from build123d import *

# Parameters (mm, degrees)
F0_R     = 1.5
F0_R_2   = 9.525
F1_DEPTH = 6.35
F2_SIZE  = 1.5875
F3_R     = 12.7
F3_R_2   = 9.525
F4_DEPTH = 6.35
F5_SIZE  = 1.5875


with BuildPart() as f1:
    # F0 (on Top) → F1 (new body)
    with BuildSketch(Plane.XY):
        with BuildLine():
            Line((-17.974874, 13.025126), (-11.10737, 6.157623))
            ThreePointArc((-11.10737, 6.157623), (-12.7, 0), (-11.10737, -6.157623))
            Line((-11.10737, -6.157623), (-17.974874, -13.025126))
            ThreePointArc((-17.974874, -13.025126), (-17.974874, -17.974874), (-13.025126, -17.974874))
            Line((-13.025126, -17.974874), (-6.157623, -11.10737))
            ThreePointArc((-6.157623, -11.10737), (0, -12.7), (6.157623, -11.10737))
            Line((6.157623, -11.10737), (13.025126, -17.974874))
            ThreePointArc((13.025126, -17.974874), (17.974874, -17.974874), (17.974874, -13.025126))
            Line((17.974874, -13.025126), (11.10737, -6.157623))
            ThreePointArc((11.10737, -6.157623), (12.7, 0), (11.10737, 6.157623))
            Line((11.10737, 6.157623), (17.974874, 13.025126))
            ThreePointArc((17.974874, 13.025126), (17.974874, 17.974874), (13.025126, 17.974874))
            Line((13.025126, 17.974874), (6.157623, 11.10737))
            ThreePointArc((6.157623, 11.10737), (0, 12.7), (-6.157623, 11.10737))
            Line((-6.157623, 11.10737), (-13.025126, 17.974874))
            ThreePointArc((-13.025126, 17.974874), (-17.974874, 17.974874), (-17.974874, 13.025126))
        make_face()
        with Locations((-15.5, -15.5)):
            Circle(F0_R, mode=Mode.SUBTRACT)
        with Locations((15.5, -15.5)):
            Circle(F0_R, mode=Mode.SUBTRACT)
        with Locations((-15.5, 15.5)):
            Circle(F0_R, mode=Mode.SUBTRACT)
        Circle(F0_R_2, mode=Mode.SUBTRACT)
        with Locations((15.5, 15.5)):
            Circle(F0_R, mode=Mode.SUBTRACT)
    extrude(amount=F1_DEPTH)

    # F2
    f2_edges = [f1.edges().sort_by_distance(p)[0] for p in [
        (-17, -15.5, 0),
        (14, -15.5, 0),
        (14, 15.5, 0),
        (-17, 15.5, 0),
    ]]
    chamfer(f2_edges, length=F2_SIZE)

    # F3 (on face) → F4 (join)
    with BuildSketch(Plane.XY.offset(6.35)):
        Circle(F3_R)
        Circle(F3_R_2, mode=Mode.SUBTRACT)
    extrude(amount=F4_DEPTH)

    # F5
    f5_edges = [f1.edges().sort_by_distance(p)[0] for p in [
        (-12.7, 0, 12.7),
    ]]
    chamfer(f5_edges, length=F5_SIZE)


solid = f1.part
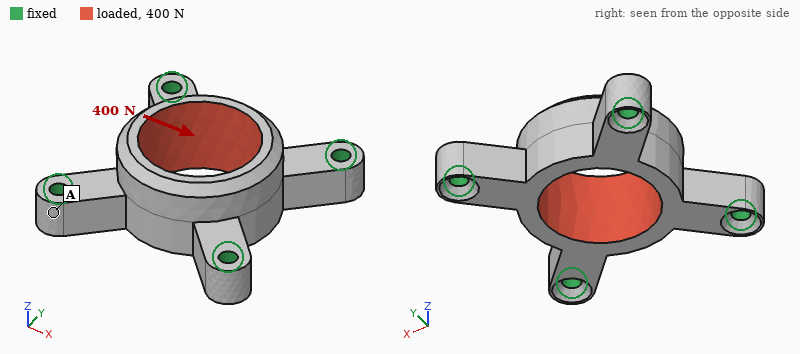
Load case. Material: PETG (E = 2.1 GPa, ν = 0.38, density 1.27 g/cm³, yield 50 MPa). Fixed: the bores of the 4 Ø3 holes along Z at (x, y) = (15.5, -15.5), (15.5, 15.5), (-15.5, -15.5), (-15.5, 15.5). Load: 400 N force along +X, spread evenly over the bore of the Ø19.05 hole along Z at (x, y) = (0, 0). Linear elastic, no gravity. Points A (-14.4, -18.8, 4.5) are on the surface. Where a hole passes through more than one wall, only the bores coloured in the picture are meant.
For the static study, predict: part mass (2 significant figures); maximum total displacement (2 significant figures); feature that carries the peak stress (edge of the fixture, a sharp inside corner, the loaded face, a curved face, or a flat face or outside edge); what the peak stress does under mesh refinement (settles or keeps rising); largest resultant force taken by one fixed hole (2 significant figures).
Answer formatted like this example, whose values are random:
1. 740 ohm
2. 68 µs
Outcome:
1. 5.9 g
2. 99 µm
3. edge of the fixture
4. keeps rising
5. 120 N
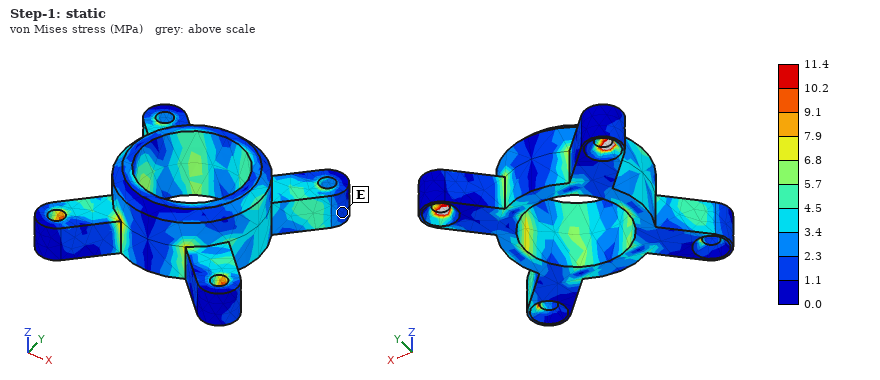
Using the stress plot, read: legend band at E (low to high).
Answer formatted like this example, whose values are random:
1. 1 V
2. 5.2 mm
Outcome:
1. 1.1 to 2.3 MPa
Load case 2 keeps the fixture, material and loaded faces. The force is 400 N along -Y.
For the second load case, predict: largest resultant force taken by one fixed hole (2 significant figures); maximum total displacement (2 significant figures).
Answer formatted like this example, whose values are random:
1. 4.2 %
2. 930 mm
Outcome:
1. 120 N
2. 99 µm
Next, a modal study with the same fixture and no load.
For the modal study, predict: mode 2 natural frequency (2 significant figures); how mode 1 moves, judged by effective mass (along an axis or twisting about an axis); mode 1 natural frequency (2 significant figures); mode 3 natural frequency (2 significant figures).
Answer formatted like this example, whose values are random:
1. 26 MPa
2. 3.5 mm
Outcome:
1. 5600 Hz
2. along Z
3. 4900 Hz
4. 6100 Hz
